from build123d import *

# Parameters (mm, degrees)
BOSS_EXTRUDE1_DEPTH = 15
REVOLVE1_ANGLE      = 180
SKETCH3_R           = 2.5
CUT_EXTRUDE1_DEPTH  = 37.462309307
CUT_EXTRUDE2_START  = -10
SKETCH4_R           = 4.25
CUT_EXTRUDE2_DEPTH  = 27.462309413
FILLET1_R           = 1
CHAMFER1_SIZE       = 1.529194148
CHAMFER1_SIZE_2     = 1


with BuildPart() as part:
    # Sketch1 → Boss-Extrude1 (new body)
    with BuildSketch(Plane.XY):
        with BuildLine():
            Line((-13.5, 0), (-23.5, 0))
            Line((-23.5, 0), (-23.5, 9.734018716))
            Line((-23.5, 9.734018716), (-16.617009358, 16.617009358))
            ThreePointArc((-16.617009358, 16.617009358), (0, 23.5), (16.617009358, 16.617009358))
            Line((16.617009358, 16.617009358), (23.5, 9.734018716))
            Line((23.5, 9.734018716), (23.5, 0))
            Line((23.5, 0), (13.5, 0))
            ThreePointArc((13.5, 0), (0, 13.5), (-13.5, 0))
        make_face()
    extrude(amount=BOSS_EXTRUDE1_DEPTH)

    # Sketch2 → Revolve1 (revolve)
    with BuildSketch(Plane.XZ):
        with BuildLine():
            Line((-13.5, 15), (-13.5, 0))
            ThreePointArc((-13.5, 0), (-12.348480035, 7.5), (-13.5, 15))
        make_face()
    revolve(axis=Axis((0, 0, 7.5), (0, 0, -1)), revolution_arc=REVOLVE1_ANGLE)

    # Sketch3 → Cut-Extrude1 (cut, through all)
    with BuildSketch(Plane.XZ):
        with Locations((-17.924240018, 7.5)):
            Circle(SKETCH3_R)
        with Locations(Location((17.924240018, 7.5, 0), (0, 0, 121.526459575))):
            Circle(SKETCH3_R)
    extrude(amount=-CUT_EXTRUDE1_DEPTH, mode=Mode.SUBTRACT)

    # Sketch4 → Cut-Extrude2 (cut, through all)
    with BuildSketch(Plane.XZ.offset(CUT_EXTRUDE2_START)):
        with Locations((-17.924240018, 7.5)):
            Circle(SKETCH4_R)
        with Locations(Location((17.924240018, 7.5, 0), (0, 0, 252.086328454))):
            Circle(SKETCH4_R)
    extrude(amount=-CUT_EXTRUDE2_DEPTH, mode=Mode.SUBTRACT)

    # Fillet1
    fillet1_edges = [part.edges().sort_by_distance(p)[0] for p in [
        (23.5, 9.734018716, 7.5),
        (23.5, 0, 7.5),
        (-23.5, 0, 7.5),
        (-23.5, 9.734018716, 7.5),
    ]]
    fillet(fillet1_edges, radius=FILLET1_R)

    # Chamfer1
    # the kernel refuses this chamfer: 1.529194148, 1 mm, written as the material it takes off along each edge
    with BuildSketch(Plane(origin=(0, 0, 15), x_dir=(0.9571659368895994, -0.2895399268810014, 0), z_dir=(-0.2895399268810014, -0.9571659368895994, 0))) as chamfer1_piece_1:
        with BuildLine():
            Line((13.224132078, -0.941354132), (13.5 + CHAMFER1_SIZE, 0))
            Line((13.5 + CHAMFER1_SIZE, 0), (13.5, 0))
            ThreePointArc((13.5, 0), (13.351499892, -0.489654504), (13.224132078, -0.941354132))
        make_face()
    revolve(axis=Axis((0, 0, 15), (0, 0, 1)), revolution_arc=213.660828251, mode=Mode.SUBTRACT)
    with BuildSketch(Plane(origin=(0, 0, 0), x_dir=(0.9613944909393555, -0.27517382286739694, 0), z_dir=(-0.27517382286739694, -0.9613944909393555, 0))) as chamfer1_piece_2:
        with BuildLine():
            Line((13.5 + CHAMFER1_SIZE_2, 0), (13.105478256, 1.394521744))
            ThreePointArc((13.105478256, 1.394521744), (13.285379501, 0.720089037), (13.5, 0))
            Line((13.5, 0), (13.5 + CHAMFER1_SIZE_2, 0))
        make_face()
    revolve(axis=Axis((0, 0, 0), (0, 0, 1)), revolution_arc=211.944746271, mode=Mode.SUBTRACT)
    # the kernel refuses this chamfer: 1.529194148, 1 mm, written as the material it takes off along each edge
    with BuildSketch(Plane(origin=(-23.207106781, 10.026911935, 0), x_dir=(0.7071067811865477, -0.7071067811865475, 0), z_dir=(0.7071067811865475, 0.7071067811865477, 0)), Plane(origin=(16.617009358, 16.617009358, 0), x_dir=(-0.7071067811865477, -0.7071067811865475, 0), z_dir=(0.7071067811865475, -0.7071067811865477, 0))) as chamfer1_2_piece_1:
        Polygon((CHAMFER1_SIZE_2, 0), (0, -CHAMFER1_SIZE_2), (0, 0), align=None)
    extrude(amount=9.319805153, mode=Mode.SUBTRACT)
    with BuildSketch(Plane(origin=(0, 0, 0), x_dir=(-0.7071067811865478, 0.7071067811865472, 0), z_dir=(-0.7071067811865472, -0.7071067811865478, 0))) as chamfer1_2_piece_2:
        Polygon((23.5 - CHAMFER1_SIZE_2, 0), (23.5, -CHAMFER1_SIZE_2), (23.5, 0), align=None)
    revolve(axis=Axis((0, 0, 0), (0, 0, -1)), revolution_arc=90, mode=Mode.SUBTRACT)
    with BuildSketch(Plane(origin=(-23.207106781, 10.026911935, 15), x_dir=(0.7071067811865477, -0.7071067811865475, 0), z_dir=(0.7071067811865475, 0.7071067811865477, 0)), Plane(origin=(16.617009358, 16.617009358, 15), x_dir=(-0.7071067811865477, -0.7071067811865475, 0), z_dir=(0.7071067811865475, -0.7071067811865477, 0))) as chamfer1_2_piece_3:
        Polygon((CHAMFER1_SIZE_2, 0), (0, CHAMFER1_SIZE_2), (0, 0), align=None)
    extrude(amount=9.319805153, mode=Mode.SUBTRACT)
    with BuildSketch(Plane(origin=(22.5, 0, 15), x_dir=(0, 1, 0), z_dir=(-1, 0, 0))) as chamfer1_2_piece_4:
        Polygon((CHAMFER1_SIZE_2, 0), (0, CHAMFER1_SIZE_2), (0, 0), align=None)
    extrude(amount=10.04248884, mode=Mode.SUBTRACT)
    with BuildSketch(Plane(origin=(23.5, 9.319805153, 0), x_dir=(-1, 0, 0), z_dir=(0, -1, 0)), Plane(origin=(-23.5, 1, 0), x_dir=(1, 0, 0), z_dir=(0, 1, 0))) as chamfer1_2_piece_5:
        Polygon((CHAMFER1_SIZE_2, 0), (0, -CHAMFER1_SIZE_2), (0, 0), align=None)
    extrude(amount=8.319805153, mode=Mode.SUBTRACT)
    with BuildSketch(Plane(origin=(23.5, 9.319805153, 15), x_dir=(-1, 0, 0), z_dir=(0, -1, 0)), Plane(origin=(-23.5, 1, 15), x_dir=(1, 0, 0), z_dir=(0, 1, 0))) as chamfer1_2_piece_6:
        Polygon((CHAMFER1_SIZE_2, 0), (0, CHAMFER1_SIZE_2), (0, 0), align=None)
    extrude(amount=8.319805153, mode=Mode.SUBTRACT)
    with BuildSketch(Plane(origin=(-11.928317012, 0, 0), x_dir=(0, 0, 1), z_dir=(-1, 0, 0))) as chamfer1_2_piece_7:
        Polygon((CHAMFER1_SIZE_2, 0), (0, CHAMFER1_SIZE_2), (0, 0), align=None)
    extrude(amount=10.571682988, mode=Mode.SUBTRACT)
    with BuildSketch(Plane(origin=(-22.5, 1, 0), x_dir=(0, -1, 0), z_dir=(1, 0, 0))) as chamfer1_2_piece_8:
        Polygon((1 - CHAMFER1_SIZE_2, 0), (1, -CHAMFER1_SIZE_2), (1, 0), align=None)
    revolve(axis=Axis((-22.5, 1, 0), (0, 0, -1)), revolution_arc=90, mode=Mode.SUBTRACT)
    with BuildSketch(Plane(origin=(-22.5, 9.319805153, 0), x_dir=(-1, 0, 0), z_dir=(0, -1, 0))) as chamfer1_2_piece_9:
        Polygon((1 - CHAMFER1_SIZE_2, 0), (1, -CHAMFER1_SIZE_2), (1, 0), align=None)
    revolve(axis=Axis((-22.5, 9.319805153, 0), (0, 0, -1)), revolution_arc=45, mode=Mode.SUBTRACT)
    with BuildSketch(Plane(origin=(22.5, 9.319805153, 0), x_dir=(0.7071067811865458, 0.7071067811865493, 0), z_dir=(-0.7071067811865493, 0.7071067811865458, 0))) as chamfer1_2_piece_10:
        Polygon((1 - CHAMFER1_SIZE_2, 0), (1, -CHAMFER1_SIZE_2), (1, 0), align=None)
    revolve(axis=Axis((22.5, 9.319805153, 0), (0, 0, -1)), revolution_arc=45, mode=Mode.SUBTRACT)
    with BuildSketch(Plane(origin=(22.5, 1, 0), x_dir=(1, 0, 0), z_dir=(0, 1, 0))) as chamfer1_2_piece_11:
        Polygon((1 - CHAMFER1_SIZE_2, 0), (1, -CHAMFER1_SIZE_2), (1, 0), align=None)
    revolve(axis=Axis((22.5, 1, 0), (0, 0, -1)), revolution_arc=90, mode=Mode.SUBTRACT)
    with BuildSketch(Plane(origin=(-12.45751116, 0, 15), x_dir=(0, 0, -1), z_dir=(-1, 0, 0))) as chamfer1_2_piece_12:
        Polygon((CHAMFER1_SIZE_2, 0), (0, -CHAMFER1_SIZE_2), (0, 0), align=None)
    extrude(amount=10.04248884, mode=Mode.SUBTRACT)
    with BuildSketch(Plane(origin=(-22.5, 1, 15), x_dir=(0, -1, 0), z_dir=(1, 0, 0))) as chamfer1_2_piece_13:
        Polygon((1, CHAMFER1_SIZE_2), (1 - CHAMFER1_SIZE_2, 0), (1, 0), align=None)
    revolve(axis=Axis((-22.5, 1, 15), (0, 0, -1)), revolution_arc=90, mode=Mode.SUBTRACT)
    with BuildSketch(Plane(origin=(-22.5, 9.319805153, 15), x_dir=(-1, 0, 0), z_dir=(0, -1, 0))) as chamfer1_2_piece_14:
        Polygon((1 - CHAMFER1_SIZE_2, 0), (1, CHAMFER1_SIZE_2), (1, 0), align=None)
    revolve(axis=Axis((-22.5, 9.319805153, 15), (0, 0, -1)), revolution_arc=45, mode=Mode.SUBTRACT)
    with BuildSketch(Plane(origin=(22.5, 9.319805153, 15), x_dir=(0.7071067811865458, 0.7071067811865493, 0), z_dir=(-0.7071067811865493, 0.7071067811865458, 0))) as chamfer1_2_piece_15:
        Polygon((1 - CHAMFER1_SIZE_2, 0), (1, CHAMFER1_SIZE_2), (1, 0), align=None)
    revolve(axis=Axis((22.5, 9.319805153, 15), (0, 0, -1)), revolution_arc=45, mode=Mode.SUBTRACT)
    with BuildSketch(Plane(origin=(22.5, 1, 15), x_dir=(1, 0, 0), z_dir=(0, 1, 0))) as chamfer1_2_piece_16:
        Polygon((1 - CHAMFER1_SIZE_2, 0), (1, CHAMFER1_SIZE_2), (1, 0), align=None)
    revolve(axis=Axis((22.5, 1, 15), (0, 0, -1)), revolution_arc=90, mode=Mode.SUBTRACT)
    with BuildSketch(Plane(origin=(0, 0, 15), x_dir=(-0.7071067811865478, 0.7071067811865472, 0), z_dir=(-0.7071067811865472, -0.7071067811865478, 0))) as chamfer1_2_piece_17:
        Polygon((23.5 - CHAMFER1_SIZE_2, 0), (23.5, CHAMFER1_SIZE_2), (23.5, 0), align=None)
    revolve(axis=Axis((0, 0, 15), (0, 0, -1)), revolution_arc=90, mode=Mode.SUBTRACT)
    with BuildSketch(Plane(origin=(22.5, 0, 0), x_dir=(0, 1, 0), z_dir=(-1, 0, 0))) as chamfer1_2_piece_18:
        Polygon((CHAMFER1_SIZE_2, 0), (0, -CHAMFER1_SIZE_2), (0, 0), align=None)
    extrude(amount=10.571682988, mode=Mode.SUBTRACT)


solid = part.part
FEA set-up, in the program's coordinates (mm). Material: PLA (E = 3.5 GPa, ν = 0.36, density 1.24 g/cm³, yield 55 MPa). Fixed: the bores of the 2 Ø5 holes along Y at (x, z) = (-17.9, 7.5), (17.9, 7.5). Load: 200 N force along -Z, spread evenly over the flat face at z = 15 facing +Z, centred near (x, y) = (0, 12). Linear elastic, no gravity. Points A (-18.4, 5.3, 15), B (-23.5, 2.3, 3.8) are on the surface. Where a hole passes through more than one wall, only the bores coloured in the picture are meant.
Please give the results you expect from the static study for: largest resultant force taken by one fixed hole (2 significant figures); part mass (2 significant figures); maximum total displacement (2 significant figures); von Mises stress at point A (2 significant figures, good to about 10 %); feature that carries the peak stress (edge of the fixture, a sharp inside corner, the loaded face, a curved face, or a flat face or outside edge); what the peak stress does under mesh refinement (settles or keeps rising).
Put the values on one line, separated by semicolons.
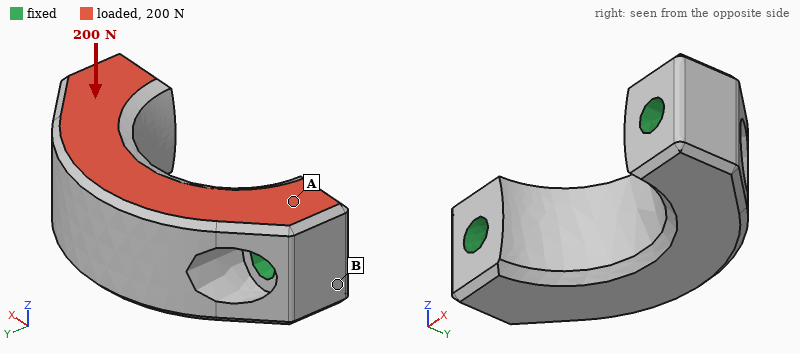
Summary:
100 N; 10 g; 28 µm; 1.4 MPa; edge of the fixture; keeps rising
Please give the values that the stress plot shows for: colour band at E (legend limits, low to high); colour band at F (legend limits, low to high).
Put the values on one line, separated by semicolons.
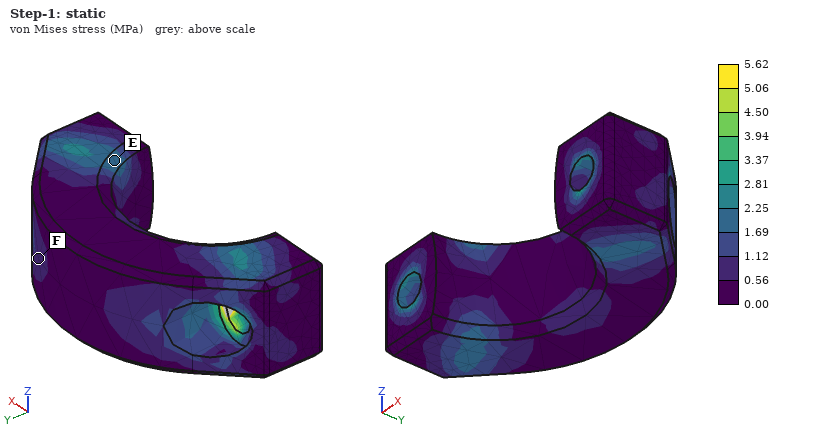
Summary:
1.69 to 2.25 MPa; 0.56 to 1.12 MPa
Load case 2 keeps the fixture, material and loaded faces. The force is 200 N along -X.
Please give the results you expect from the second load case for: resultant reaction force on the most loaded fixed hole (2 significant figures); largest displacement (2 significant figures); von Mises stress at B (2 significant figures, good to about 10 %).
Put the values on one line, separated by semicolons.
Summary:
110 N; 10 µm; 0.26 MPa
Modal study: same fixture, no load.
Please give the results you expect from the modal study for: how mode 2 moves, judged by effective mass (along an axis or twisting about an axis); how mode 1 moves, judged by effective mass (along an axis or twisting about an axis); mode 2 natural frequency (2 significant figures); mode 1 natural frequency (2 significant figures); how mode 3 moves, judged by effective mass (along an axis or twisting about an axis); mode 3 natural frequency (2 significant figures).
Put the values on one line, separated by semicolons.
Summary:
along X; along Z; 11 kHz; 5100 Hz; along Y; 11 kHz
